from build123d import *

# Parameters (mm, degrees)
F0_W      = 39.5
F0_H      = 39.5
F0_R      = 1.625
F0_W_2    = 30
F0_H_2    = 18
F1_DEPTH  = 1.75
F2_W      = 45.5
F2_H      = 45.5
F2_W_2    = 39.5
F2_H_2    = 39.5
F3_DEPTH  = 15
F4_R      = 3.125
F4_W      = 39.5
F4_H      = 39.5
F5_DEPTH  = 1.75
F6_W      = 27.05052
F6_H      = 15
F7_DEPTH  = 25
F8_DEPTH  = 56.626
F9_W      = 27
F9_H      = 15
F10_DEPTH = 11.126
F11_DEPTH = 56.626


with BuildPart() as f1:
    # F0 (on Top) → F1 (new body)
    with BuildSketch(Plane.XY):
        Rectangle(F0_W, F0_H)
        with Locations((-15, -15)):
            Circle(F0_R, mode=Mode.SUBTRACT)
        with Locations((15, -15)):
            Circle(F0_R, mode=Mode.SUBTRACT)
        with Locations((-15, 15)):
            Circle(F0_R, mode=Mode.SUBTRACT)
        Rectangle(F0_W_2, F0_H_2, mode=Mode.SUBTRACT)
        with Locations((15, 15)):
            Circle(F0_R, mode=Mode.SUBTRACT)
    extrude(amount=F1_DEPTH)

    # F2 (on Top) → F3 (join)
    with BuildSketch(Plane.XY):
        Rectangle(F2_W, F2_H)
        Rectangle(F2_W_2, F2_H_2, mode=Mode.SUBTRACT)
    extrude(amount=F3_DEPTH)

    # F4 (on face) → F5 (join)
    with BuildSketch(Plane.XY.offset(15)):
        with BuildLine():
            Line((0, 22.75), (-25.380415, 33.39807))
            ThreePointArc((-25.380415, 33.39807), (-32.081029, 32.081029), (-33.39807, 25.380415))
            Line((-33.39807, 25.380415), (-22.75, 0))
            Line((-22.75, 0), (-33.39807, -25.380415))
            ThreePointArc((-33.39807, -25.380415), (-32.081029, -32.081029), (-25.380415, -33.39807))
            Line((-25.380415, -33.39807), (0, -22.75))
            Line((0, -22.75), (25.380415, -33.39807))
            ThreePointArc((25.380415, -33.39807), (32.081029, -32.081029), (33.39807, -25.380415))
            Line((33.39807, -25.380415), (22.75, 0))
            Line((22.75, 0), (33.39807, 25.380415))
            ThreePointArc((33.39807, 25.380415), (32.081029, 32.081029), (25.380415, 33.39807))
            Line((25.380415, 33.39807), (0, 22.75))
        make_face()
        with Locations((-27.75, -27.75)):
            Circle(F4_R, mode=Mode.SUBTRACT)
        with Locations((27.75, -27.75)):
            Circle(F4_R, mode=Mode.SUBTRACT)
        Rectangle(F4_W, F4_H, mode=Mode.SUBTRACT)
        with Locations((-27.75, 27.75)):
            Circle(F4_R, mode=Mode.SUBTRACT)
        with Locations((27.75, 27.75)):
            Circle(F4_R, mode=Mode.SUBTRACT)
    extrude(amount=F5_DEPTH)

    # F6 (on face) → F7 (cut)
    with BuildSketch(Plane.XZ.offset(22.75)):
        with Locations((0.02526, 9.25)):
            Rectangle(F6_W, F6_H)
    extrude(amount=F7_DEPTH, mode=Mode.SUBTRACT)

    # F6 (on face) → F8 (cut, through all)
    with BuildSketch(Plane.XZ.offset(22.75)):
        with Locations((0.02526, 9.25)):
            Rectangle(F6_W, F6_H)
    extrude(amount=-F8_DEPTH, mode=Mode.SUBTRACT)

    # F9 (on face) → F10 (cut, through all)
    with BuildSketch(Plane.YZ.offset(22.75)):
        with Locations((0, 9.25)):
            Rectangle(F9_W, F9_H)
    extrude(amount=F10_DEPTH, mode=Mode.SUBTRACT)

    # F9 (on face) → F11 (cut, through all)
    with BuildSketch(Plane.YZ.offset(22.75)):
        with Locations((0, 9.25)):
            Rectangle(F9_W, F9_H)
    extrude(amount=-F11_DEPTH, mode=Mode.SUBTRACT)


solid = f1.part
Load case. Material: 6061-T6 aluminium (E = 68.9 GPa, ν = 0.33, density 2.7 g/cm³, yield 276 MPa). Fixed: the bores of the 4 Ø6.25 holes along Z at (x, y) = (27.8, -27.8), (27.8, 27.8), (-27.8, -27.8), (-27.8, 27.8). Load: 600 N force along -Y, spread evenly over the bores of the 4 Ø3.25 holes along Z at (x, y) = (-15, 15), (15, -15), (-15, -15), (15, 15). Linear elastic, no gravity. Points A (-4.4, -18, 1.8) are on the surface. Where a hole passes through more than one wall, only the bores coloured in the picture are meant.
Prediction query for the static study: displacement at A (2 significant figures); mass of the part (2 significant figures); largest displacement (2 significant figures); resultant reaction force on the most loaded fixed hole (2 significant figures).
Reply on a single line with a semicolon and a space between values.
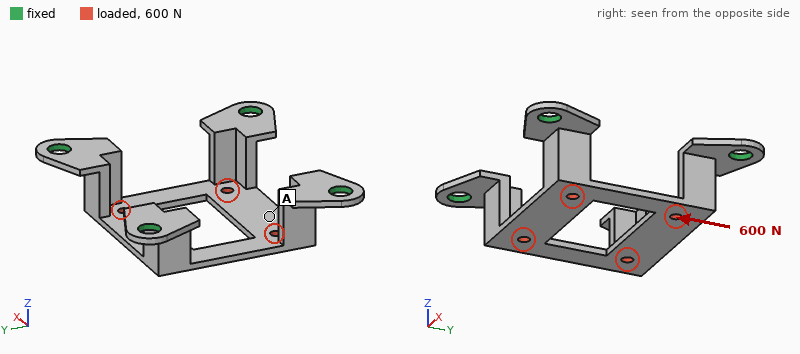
0.15 mm; 19 g; 0.19 mm; 160 N
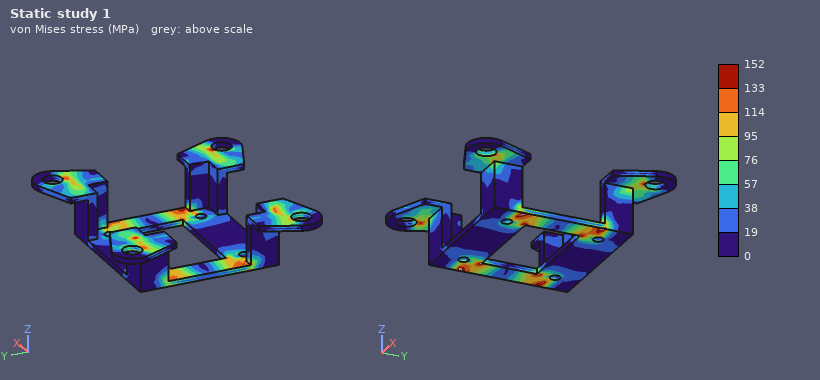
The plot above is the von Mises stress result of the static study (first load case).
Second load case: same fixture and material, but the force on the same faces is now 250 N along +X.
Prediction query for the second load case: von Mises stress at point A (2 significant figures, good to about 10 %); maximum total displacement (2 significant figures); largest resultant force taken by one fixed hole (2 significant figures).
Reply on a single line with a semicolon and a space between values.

17 MPa; 69 µm; 67 N
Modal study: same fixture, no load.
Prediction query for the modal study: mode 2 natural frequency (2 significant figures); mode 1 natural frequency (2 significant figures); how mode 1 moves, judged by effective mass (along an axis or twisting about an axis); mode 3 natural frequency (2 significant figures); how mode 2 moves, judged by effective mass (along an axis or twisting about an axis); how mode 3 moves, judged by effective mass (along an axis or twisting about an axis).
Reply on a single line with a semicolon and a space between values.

3200 Hz; 2900 Hz; along Y; 4700 Hz; along X; twisting about Z
